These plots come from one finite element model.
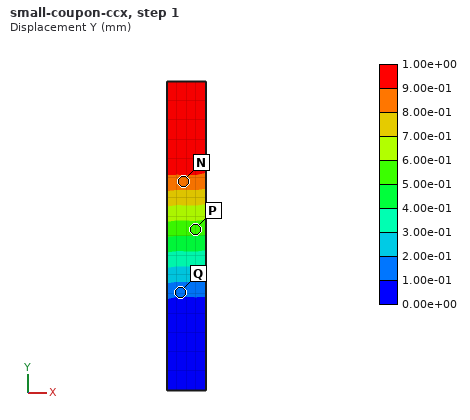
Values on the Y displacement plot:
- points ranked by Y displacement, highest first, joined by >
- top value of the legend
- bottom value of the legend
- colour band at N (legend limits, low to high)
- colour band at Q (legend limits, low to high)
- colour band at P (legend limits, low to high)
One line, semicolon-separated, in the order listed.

N > P > Q; 1.00e+00 mm; 0.00e+00 mm; 8.00e-01 to 9.00e-01 mm; 1.00e-01 to 2.00e-01 mm; 5.00e-01 to 6.00e-01 mm
